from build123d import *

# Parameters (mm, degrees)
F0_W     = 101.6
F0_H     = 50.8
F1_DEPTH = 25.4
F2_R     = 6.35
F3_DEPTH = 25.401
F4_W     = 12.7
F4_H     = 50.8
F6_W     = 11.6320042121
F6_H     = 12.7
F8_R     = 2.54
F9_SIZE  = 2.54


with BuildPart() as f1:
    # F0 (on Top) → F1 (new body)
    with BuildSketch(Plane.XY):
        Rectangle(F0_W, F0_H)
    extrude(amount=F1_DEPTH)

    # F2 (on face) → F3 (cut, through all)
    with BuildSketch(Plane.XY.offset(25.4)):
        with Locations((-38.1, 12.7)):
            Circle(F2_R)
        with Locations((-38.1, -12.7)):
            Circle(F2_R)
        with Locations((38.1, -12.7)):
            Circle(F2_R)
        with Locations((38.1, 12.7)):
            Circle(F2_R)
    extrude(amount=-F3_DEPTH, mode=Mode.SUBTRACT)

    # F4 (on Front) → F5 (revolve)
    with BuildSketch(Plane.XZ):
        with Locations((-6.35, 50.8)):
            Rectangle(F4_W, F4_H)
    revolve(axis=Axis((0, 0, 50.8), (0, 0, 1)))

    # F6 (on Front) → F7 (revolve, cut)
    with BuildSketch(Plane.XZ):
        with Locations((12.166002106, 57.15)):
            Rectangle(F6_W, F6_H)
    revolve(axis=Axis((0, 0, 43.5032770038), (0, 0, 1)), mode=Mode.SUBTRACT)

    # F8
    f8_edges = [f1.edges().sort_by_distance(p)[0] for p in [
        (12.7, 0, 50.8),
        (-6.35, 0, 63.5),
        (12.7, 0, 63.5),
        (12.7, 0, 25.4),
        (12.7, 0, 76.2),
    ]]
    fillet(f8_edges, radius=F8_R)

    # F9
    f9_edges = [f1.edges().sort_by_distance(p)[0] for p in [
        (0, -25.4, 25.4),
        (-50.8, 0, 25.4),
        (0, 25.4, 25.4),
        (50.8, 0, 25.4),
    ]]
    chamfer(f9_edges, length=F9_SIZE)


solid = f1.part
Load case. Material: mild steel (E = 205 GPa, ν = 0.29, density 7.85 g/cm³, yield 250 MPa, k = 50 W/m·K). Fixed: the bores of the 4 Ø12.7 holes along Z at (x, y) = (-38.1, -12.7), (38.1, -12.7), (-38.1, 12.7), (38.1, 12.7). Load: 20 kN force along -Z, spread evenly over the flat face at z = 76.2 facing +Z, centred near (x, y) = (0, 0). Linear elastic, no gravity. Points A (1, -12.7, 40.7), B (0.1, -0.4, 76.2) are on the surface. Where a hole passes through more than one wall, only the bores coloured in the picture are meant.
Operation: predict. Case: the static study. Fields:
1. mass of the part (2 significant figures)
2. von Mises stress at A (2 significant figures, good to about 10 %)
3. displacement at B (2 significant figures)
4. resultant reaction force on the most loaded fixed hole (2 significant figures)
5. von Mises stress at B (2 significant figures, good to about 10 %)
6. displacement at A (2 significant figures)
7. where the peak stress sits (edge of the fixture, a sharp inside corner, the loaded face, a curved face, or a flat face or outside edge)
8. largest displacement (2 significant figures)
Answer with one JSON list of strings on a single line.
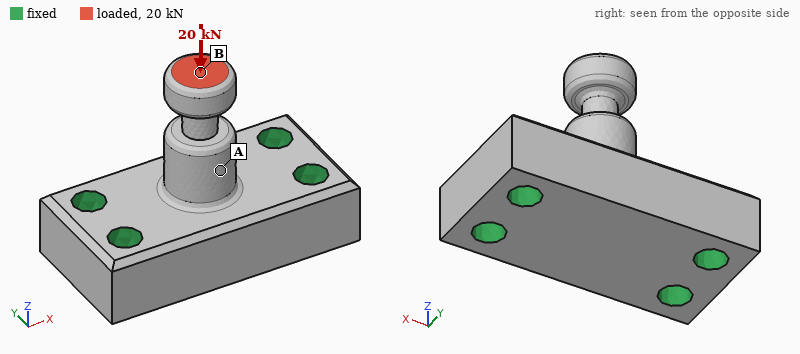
["1.1 kg", "30 MPa", "27 µm", "5.1 kN", "62 MPa", "8.2 µm", "a curved face", "27 µm"]
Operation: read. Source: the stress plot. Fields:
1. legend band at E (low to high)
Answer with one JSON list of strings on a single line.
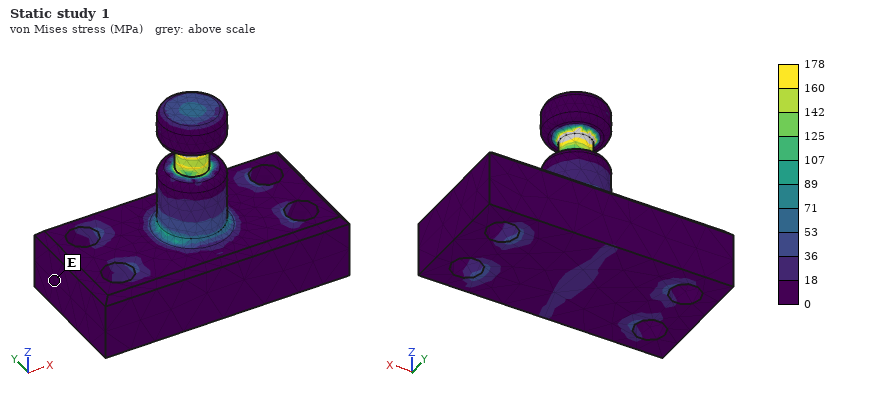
["0 to 18 MPa"]
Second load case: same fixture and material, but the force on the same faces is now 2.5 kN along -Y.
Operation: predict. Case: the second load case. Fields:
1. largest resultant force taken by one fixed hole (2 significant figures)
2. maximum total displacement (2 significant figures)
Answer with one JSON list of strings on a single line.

["2.1 kN", "0.11 mm"]
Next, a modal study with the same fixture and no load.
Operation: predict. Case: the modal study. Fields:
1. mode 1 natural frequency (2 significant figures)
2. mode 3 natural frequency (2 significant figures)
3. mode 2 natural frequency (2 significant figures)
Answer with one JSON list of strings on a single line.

["4100 Hz", "8800 Hz", "4300 Hz"]
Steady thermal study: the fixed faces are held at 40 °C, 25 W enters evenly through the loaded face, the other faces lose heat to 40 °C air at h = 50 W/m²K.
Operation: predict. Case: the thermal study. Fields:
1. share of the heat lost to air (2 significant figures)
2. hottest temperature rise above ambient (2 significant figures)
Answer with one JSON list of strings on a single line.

["36 %", "85 K"]
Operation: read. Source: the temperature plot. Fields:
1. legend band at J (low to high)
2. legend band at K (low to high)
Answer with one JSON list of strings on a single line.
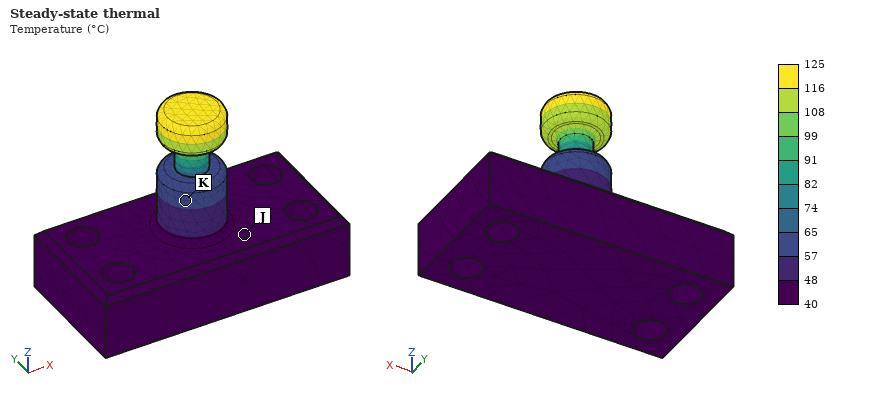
["40 to 48 °C", "57 to 65 °C"]
